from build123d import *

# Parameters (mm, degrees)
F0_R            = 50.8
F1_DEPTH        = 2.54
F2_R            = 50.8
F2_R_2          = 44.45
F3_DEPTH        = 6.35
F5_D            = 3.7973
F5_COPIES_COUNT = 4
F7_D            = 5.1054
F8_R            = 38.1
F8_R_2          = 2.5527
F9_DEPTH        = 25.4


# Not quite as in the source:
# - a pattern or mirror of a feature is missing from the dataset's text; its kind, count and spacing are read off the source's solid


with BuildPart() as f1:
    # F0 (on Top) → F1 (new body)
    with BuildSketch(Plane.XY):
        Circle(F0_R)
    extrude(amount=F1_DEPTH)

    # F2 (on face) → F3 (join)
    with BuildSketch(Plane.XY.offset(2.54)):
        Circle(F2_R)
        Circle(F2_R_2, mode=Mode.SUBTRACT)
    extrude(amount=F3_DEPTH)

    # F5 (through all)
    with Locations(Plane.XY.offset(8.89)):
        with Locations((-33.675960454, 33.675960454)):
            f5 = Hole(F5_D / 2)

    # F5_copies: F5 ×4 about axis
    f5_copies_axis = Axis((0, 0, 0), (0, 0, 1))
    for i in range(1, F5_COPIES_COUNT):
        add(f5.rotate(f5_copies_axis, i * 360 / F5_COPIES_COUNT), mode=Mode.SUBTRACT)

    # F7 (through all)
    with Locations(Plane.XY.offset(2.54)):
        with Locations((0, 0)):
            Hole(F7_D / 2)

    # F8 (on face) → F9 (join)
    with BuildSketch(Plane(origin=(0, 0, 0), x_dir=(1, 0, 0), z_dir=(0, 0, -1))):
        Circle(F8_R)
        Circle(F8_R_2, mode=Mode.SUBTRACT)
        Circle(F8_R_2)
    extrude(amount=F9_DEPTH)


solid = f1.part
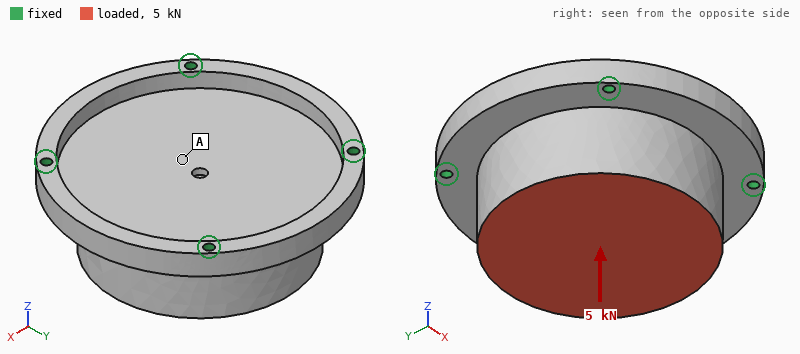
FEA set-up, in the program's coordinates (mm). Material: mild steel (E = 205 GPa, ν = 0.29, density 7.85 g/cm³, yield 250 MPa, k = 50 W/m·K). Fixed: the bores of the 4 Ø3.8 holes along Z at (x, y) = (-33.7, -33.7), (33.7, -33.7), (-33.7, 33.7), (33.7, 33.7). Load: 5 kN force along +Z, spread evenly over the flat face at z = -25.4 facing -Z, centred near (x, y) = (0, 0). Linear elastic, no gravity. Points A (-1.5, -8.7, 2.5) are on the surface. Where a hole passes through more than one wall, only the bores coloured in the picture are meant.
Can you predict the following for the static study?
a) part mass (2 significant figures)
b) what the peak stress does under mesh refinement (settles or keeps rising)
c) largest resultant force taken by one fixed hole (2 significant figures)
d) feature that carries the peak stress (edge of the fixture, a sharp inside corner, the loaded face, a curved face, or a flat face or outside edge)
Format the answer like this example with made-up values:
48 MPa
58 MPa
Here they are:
1.2 kg
keeps rising
1.5 kN
edge of the fixture
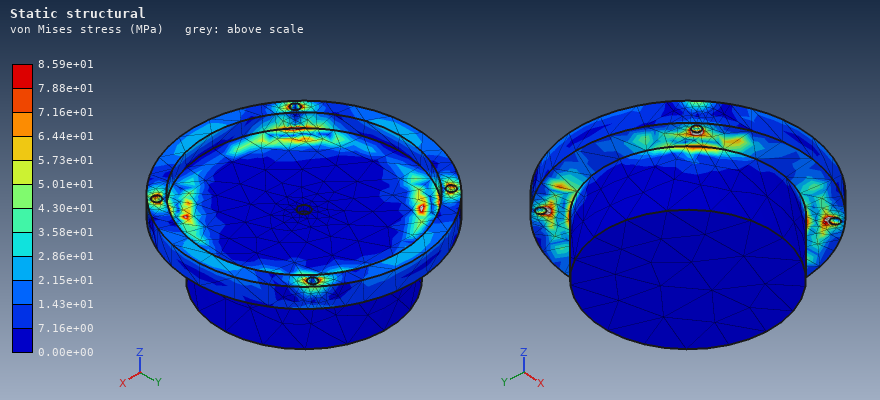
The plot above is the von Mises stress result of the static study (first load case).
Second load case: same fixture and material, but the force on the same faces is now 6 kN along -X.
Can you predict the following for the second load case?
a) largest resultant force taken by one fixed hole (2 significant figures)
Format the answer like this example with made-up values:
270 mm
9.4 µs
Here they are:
2.0 kN
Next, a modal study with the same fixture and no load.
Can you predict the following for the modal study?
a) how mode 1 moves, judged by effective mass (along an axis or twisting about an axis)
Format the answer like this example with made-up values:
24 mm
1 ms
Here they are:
along Z
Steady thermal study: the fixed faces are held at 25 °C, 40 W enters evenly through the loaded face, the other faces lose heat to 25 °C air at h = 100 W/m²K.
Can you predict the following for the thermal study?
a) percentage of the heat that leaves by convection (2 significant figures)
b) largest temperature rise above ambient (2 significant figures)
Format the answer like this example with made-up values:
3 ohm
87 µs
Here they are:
58 %
18 K
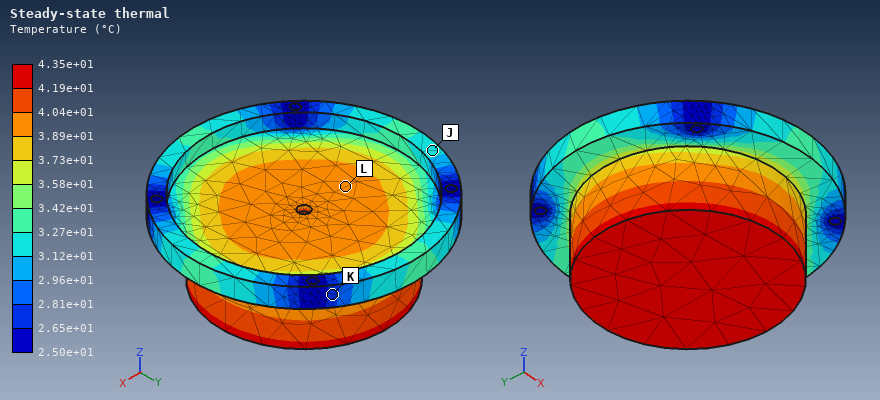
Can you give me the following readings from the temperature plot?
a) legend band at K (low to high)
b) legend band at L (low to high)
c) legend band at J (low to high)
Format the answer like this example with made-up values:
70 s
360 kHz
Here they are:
2.65e+01 to 2.81e+01 °C
3.89e+01 to 4.04e+01 °C
3.12e+01 to 3.27e+01 °C
